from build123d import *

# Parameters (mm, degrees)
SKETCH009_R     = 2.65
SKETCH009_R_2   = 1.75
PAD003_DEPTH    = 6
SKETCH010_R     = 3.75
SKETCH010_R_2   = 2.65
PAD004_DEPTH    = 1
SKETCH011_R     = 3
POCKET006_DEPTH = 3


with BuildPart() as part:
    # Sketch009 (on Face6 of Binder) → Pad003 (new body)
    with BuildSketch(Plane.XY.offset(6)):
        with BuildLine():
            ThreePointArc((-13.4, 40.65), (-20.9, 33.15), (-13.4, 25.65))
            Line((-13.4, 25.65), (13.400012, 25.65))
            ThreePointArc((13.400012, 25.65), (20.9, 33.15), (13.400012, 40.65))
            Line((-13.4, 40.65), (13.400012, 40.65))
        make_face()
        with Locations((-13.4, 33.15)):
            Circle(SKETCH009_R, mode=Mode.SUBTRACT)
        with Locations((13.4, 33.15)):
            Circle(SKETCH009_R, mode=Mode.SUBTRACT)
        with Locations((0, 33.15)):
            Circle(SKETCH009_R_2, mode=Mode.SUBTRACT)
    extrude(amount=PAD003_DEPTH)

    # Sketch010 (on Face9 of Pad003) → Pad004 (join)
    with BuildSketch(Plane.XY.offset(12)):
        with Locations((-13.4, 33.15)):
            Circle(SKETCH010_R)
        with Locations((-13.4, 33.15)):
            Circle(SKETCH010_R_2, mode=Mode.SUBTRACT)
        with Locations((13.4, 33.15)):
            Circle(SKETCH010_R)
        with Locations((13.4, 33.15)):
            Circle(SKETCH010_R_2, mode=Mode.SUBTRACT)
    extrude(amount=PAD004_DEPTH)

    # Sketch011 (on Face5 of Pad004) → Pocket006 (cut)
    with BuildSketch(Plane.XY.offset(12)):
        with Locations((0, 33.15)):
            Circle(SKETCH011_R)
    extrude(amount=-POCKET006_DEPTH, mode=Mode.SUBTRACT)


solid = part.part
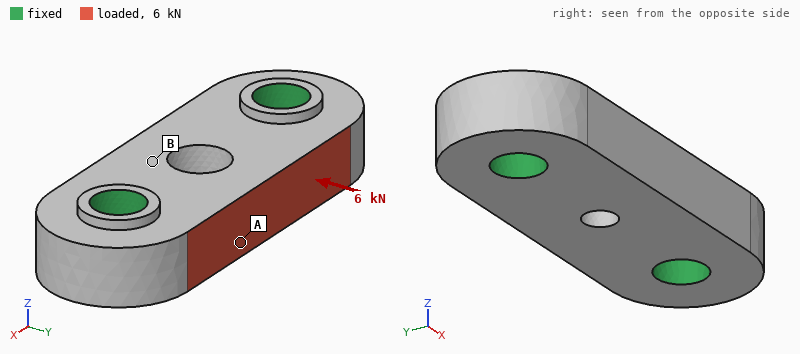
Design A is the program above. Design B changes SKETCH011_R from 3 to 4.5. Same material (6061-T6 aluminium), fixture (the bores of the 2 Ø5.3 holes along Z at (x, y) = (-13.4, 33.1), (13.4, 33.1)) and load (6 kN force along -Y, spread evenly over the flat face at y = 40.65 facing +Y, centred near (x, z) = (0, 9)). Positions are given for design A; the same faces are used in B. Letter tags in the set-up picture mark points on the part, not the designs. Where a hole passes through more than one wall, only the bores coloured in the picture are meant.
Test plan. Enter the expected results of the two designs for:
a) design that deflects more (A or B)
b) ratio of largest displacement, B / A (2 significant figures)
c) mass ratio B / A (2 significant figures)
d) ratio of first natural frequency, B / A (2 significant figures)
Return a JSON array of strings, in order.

["B", "1.2", "0.97", "1.0"]
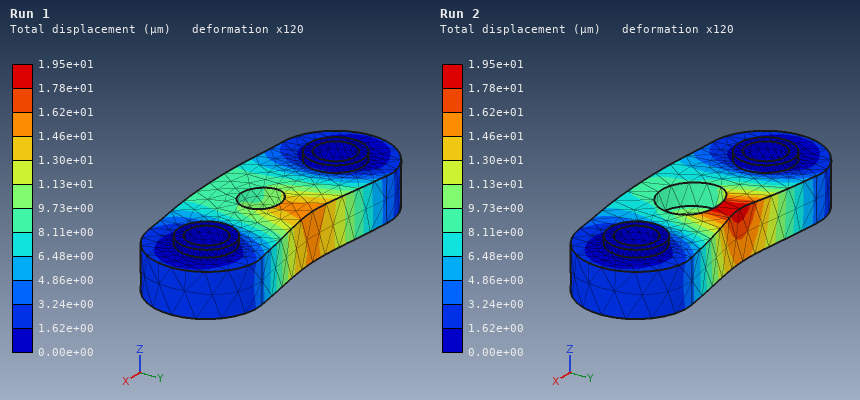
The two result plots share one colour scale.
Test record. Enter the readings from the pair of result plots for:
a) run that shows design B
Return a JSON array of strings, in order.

["Run 2"]
